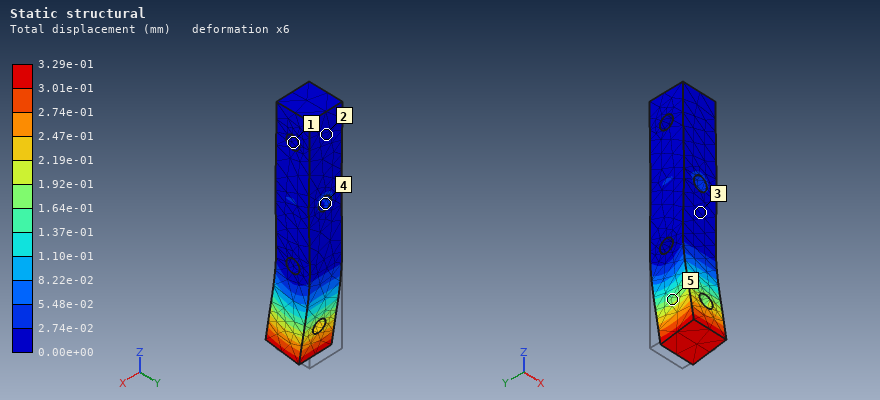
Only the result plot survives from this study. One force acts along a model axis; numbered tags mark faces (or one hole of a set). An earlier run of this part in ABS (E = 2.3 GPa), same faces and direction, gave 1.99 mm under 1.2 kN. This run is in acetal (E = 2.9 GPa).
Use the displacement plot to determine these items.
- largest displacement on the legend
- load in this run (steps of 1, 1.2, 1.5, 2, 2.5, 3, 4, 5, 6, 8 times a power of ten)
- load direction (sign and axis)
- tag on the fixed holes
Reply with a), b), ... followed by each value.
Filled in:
a) 3.29e-01 mm
b) 250 N
c) -Y
d) 1
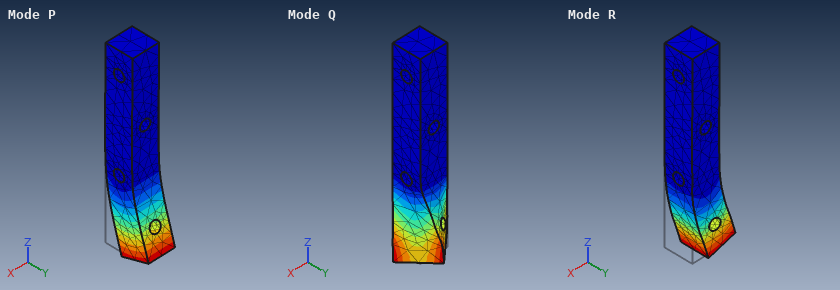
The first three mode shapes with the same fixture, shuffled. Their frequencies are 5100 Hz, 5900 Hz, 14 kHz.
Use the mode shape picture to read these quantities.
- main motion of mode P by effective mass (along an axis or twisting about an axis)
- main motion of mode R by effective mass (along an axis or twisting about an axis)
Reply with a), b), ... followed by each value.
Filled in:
a) along Y
b) along X
